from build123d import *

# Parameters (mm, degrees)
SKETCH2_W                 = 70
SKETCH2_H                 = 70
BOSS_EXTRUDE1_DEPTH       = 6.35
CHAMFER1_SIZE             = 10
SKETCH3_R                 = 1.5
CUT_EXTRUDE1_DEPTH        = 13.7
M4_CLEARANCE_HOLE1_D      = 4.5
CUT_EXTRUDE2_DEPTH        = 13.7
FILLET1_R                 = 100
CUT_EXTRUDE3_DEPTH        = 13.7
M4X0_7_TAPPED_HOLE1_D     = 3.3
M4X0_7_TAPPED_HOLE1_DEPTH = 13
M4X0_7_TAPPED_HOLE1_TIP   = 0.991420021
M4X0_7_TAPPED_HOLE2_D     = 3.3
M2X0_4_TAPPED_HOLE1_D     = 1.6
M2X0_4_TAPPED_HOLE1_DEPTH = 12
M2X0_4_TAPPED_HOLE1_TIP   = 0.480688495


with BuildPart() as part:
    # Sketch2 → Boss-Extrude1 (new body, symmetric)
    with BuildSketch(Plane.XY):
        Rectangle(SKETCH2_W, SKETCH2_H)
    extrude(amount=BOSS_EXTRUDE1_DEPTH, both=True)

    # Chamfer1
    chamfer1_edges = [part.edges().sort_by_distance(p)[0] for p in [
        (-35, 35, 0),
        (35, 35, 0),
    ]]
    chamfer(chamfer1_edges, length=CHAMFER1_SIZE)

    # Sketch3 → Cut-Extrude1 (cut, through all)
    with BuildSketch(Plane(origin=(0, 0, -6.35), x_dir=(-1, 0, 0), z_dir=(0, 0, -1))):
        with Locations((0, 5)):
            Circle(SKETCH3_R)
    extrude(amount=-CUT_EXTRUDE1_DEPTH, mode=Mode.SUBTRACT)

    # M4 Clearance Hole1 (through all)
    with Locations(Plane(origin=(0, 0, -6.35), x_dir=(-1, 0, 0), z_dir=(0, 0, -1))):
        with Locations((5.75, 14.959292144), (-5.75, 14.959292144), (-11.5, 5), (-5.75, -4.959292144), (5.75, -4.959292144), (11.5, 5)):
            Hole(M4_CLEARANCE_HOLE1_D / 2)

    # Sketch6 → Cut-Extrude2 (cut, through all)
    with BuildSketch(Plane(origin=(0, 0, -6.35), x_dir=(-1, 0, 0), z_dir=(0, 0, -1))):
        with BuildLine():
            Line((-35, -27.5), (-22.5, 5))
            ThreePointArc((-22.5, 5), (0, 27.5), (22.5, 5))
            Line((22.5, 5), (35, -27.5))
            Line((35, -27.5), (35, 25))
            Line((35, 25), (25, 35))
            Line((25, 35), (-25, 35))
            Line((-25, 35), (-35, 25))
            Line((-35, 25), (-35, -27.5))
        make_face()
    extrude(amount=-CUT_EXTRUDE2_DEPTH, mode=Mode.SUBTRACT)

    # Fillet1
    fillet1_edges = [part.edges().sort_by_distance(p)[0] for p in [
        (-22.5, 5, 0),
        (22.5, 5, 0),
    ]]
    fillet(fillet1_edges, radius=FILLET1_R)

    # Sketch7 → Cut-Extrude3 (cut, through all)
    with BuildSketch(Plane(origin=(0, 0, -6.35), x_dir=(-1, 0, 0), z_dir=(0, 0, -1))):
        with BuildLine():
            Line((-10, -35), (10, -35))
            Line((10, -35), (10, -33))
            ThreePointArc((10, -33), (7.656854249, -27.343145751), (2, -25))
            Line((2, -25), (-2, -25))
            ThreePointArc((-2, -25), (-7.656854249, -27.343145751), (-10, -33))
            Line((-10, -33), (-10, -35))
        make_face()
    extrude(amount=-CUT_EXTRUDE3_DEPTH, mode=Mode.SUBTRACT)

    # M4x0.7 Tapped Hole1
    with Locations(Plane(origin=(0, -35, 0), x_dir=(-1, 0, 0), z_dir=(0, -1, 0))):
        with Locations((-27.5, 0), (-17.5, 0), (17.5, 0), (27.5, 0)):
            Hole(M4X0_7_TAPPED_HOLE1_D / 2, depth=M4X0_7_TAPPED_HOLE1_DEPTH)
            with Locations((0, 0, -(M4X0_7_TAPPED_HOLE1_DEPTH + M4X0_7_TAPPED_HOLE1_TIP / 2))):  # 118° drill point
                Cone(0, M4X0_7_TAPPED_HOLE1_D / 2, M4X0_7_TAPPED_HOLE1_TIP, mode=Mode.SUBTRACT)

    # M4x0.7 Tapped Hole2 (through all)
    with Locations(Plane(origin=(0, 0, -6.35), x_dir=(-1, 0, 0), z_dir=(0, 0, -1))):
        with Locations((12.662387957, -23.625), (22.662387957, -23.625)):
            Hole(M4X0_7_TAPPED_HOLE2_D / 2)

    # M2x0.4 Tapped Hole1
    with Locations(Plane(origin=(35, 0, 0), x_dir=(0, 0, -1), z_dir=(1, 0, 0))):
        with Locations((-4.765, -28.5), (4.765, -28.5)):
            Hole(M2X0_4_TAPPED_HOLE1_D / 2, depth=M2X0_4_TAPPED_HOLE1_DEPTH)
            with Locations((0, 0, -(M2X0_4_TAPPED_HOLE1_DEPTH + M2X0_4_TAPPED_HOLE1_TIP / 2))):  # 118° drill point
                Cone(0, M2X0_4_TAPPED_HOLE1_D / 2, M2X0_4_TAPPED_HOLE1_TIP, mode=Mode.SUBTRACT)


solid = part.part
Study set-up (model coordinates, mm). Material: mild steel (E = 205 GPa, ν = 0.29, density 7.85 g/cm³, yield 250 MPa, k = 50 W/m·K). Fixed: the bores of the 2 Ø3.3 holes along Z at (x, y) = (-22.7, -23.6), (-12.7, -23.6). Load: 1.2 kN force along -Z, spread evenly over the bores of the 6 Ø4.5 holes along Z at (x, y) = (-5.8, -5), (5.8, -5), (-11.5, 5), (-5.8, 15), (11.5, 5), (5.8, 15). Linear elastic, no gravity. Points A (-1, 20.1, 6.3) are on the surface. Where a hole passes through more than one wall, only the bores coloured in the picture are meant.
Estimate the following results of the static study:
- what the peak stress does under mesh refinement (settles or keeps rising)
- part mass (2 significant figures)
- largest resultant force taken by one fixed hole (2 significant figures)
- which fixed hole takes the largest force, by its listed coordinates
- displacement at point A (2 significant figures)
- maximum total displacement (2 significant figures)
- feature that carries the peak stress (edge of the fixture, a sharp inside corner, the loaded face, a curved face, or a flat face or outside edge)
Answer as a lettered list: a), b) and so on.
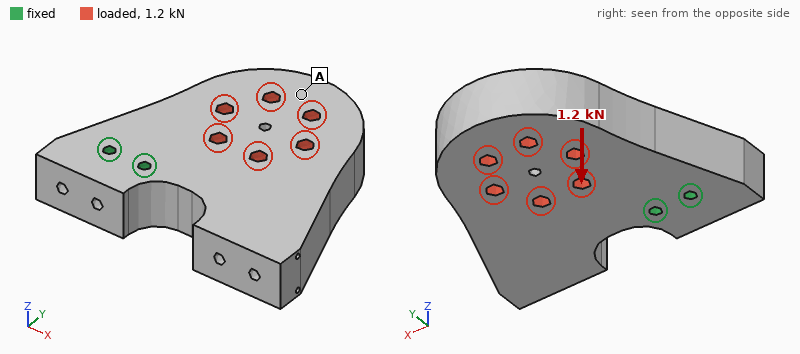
a) keeps rising
b) 290 g
c) 1.3 kN
d) (-12.7, -23.6)
e) 26 µm
f) 32 µm
g) edge of the fixture
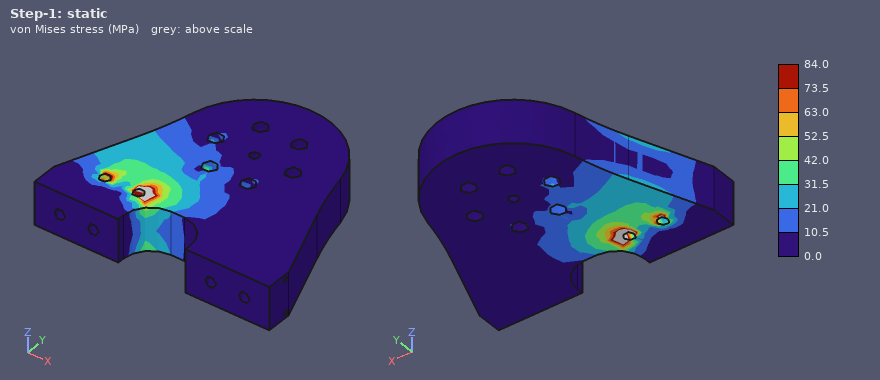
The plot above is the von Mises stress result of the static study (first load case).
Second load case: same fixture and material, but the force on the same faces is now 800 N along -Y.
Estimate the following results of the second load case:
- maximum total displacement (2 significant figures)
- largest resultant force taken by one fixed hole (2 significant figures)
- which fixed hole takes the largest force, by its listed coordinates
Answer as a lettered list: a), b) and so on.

a) 4.7 µm
b) 1.5 kN
c) (-12.7, -23.6)
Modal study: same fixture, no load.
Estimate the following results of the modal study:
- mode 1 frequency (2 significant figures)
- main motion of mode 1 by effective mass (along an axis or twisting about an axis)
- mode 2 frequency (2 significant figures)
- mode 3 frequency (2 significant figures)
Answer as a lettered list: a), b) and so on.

a) 2900 Hz
b) along Z
c) 3700 Hz
d) 4100 Hz
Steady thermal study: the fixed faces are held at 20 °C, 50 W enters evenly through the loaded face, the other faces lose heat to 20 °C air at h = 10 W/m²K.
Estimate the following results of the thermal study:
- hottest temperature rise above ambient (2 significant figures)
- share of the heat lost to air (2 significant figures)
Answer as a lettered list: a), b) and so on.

a) 75 K
b) 8.5 %
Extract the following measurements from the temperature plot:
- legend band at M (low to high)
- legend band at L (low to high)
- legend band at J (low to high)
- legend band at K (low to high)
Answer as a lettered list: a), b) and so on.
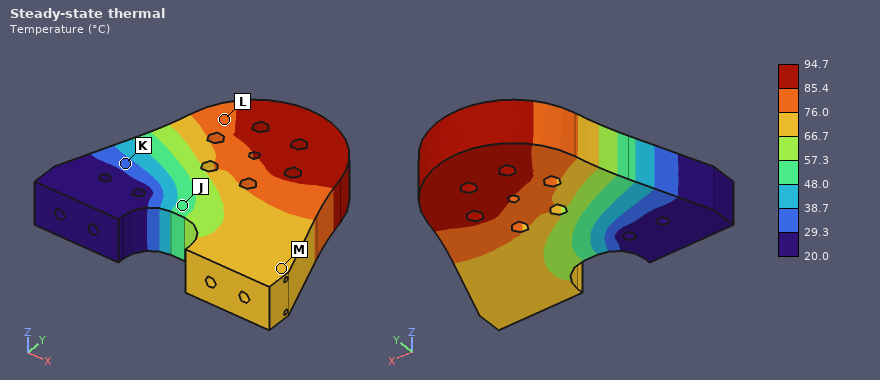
a) 66.7 to 76.0 °C
b) 76.0 to 85.4 °C
c) 48.0 to 57.3 °C
d) 29.3 to 38.7 °C
